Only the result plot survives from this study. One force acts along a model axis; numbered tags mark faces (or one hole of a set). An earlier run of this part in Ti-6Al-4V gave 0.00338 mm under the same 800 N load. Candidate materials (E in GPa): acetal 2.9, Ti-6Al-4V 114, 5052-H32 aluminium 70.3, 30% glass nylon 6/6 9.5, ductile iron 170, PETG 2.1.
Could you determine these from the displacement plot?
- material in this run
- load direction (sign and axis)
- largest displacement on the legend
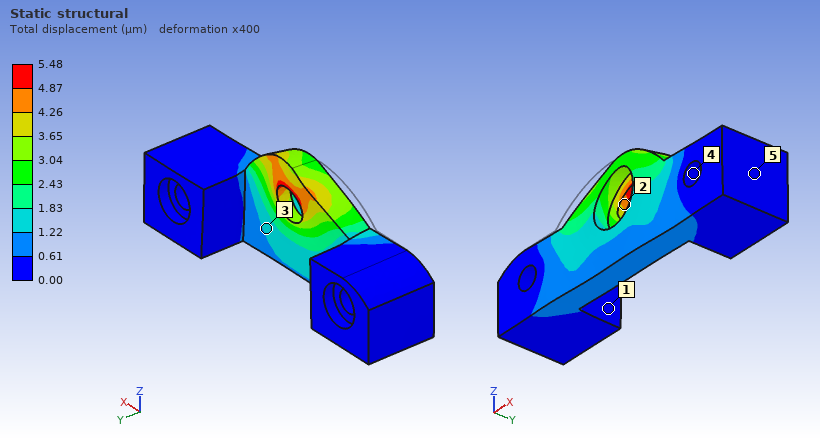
5052-H32 aluminium
+X
5.48 µm
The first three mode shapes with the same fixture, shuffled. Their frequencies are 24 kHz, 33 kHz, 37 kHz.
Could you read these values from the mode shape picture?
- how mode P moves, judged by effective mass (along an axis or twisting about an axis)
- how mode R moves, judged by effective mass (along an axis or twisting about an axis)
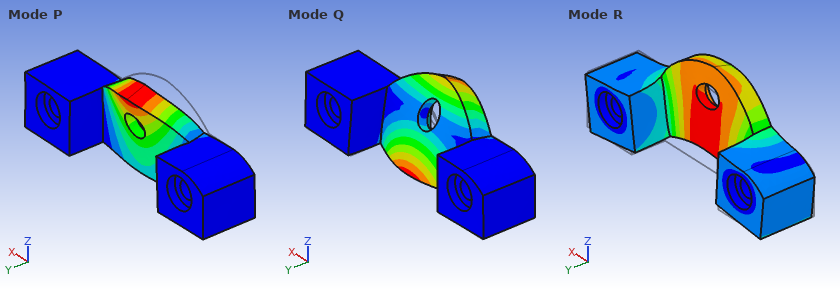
along Y
along Z
